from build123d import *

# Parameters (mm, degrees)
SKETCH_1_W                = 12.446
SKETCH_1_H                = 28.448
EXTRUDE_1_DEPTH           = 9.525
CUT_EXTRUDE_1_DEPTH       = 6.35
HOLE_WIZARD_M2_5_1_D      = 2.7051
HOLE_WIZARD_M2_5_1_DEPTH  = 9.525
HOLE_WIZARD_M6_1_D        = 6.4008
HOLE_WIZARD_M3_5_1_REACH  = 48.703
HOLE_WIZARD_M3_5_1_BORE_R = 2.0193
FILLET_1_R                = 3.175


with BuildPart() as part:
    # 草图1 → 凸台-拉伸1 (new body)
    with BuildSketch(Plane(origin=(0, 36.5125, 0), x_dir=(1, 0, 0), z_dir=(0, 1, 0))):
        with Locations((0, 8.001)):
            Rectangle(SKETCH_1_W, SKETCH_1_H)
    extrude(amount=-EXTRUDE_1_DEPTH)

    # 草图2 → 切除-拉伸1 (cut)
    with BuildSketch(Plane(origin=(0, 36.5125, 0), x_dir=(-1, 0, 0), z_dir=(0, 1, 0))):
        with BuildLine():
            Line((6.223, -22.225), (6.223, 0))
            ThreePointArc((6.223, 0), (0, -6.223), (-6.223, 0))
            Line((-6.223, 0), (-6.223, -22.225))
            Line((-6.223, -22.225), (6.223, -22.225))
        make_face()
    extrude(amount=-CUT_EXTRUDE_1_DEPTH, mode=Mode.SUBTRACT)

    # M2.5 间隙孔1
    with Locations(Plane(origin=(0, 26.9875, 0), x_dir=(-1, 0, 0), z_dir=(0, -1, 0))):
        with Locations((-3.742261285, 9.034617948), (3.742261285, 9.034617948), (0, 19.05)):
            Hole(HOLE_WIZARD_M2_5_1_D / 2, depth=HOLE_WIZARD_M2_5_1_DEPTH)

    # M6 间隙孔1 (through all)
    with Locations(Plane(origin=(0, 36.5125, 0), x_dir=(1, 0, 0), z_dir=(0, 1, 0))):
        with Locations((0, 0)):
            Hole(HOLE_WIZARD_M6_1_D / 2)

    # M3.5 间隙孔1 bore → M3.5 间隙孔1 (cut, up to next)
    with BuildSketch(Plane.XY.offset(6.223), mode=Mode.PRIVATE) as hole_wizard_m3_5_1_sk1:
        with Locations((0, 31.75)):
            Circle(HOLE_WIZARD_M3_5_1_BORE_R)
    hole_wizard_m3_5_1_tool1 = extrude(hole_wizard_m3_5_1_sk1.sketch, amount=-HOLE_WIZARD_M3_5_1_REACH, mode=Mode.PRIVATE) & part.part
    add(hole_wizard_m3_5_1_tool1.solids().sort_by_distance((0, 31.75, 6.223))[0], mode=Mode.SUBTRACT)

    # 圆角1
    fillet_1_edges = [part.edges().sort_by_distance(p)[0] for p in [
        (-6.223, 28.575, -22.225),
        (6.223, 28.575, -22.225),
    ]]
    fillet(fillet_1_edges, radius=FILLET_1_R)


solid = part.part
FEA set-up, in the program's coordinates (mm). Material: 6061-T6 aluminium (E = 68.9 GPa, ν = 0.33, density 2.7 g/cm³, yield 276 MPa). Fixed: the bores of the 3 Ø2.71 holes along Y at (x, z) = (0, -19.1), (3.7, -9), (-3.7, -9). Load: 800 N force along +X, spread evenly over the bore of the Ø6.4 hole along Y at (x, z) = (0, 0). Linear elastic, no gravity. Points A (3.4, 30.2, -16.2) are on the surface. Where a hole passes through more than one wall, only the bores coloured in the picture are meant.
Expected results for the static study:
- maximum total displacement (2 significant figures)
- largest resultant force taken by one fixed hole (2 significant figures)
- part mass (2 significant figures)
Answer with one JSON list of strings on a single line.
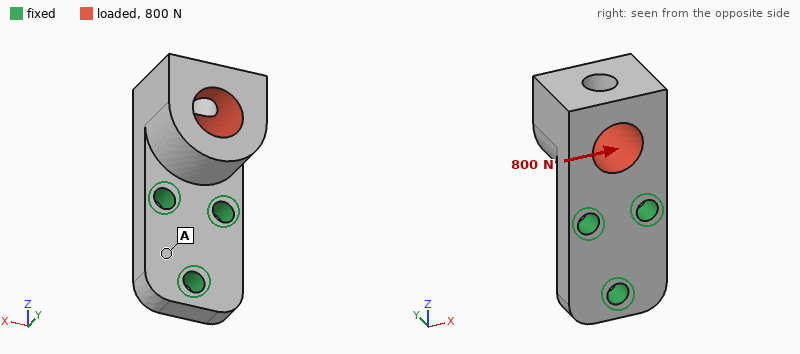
["33 µm", "870 N", "4.3 g"]
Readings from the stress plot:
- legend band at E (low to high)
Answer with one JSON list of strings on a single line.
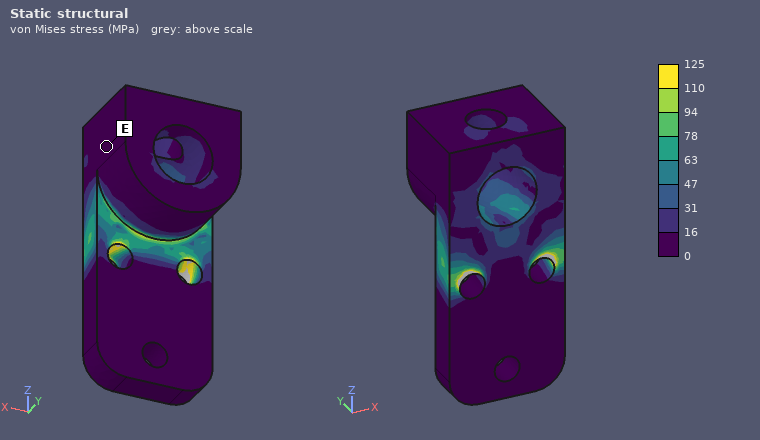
["0 to 16 MPa"]
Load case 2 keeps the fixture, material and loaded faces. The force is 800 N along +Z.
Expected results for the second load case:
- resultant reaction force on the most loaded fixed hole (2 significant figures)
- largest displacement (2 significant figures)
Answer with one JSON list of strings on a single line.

["400 N", "75 µm"]
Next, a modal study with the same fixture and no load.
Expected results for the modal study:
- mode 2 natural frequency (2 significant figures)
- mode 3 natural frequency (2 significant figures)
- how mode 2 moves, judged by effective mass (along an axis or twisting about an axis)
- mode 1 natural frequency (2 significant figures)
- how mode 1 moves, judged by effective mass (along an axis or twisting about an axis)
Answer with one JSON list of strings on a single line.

["18 kHz", "22 kHz", "along X", "7700 Hz", "along Y"]
